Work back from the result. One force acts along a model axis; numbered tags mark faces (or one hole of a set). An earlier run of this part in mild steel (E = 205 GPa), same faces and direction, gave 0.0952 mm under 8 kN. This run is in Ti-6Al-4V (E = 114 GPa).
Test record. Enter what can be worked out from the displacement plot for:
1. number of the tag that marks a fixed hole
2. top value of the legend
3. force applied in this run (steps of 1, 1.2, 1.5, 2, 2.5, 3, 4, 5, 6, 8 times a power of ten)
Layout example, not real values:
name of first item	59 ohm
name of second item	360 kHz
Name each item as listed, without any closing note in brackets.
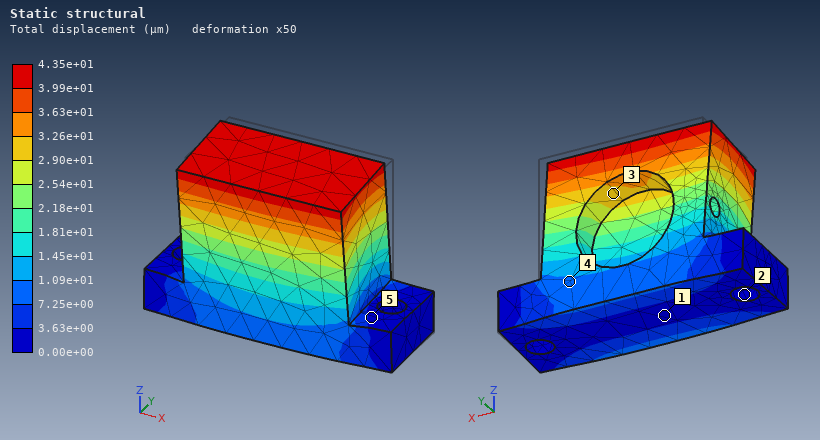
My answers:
number of the tag that marks a fixed hole	2
top value of the legend	4.35e+01 µm
force applied in this run	2 kN
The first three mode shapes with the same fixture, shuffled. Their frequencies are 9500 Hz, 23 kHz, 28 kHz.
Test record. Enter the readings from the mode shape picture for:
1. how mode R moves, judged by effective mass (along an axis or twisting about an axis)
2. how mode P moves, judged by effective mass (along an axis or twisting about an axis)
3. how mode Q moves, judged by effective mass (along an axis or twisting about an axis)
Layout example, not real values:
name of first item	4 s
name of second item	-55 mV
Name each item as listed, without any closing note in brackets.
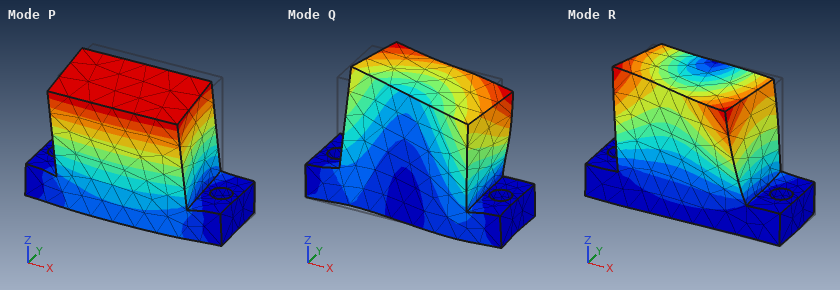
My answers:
how mode R moves, judged by effective mass	along X
how mode P moves, judged by effective mass	along Y
how mode Q moves, judged by effective mass	along X
